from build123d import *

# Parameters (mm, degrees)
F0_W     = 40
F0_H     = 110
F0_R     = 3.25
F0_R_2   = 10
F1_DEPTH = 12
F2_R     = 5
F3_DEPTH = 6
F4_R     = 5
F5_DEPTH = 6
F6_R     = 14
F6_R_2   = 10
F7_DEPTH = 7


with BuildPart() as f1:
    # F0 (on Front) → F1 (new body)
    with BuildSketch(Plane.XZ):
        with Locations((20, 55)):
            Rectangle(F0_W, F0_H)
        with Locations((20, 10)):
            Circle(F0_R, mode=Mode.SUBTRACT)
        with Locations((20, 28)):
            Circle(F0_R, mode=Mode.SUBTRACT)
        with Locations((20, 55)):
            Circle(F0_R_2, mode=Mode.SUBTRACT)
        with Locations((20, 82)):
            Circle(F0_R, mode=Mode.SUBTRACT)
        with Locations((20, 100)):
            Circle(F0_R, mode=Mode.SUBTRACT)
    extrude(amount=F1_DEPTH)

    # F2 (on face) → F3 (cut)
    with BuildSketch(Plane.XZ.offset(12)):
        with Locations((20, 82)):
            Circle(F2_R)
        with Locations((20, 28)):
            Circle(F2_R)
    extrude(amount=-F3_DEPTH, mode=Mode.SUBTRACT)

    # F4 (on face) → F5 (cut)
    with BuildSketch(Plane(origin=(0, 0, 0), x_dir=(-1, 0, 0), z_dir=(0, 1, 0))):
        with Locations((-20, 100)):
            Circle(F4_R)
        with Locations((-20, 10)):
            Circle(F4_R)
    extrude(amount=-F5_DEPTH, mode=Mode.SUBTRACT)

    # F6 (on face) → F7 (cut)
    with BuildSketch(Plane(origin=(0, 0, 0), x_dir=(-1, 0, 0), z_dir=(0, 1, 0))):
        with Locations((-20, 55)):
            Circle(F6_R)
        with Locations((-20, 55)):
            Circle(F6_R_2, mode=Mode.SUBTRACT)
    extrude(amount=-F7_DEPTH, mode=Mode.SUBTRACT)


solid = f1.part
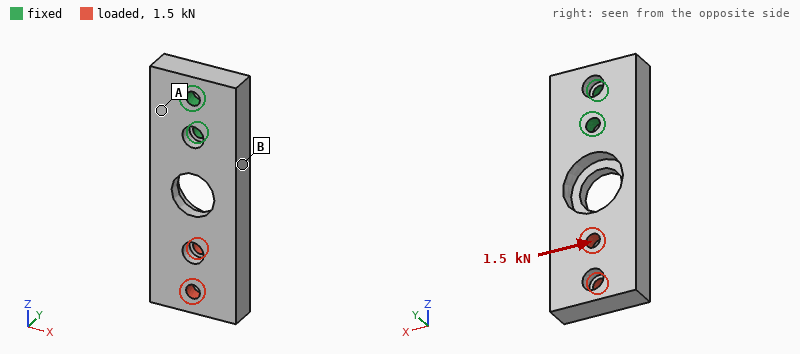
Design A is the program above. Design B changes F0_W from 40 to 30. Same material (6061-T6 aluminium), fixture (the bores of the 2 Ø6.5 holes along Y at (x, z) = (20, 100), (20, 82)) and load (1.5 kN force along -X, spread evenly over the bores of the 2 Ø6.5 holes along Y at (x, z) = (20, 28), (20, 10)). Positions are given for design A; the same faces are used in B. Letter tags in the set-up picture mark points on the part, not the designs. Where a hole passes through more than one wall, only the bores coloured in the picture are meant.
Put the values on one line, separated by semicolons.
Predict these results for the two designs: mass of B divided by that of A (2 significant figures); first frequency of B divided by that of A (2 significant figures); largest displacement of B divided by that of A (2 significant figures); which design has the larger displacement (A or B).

0.70; 0.82; 2.2; B
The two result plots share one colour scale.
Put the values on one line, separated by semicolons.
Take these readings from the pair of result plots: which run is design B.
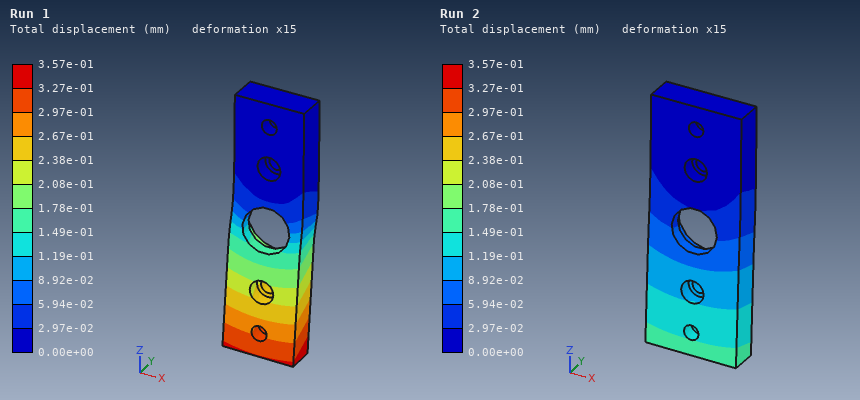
Run 1
